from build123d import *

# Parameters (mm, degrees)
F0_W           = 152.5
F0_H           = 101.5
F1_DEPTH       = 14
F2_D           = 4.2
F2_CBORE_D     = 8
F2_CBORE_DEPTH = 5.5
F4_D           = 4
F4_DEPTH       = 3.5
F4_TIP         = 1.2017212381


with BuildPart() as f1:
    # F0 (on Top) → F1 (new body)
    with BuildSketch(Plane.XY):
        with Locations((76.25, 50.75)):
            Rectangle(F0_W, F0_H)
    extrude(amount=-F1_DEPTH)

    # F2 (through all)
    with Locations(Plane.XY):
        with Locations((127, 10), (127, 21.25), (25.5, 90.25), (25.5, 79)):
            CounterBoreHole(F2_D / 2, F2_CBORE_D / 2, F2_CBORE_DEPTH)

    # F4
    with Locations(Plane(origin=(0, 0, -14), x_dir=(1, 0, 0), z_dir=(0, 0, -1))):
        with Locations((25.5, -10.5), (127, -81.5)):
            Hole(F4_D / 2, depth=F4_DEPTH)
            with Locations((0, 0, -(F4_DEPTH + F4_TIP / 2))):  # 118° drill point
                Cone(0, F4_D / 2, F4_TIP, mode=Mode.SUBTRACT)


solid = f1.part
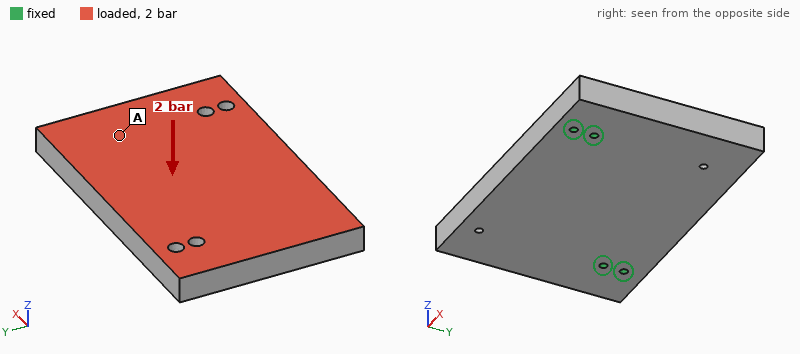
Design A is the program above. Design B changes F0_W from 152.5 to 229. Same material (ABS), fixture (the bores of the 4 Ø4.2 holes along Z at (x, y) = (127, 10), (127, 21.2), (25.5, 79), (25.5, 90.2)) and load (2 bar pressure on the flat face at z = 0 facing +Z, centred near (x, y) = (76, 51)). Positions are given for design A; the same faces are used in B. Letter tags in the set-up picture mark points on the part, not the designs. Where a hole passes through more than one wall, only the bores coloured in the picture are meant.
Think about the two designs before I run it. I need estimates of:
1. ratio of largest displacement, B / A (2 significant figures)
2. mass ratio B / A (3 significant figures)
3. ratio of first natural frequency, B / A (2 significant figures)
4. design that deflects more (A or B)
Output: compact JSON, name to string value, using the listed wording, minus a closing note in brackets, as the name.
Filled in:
{"ratio of largest displacement, B / A": "2.6", "mass ratio B / A": "1.51", "ratio of first natural frequency, B / A": "0.68", "design that deflects more": "B"}
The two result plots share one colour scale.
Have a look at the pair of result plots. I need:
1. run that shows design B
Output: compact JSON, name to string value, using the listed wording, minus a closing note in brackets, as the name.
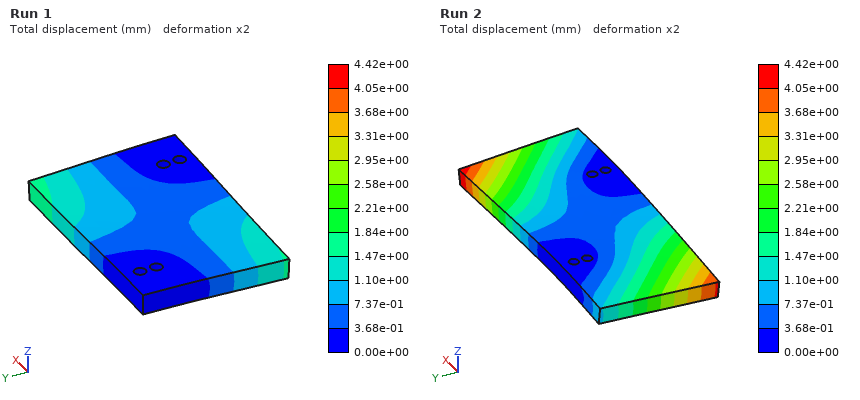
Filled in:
{"run that shows design B": "Run 2"}
